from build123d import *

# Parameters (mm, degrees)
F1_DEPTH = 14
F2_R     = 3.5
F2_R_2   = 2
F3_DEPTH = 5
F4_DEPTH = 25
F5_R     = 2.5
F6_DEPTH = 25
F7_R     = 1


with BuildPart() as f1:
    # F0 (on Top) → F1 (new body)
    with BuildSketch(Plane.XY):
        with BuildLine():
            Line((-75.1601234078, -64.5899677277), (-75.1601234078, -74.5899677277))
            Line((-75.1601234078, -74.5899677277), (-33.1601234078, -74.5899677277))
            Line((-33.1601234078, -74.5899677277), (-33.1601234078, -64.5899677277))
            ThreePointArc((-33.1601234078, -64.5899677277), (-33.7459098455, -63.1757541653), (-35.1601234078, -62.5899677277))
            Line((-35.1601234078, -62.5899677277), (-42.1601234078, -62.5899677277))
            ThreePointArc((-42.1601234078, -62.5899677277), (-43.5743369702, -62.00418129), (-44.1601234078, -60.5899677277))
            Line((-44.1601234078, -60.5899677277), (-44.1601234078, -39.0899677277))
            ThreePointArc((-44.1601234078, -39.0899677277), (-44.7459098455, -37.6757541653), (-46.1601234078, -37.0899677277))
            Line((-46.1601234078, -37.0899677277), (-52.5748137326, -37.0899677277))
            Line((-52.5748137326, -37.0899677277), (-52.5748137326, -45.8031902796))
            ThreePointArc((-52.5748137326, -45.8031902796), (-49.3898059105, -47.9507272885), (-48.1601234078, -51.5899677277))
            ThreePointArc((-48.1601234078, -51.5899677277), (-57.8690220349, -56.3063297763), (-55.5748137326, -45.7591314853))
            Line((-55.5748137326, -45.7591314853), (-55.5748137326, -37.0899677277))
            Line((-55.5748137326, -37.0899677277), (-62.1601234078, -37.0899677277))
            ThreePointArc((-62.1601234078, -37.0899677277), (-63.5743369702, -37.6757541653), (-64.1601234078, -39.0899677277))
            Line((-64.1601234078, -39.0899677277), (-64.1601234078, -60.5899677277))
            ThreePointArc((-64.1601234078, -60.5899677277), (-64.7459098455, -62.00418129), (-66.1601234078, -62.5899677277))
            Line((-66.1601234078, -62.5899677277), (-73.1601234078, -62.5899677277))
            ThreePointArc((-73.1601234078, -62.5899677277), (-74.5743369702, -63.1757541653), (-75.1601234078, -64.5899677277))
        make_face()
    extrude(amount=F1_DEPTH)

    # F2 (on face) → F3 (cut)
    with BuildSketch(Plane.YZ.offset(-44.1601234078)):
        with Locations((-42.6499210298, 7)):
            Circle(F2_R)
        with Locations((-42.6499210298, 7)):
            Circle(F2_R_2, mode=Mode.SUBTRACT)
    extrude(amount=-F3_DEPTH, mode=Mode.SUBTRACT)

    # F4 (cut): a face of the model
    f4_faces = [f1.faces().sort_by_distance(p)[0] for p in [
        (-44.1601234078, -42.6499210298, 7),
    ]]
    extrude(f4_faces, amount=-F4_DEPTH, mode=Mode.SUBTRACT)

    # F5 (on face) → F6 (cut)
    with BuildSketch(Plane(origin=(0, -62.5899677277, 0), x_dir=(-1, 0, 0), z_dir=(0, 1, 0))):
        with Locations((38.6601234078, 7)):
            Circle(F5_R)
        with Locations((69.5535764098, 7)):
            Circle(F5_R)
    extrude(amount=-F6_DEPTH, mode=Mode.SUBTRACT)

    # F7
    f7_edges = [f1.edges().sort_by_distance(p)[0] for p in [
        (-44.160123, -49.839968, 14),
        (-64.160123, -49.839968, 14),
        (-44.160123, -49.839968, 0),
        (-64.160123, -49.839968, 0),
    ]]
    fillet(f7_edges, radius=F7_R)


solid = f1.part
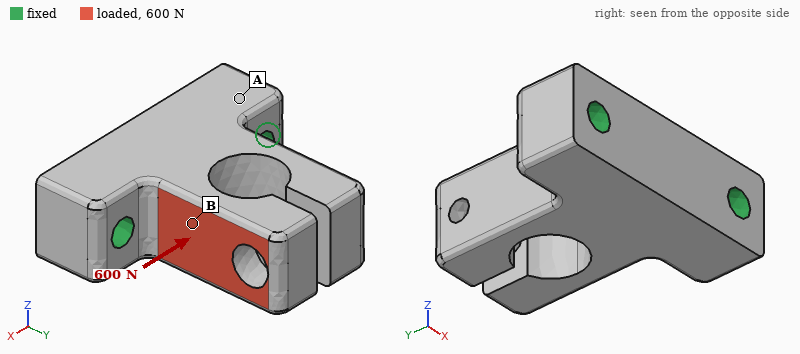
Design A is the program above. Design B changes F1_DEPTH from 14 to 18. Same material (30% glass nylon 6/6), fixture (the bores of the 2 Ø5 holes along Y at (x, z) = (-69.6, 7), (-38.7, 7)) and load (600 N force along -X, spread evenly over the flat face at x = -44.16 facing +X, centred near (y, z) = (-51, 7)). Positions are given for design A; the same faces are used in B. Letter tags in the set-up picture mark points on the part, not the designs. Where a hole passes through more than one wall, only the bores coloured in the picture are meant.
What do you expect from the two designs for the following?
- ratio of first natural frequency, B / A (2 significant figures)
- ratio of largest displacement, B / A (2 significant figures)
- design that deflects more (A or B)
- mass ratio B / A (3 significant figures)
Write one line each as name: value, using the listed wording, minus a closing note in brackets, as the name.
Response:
ratio of first natural frequency, B / A: 1.00
ratio of largest displacement, B / A: 0.83
design that deflects more: A
mass ratio B / A: 1.31
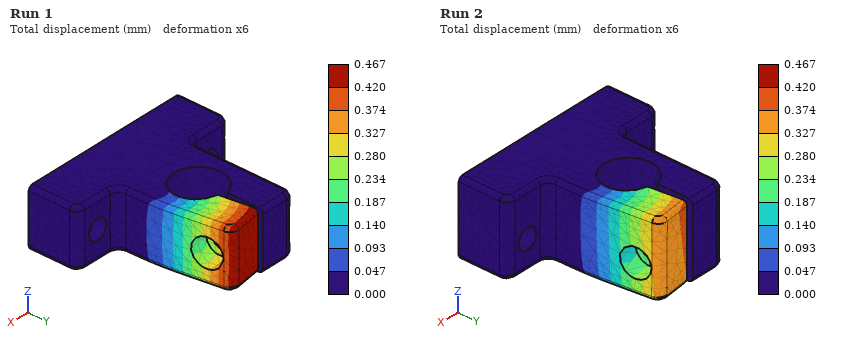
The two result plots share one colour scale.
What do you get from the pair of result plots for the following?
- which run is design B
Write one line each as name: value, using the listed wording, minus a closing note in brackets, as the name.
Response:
which run is design B: Run 2
